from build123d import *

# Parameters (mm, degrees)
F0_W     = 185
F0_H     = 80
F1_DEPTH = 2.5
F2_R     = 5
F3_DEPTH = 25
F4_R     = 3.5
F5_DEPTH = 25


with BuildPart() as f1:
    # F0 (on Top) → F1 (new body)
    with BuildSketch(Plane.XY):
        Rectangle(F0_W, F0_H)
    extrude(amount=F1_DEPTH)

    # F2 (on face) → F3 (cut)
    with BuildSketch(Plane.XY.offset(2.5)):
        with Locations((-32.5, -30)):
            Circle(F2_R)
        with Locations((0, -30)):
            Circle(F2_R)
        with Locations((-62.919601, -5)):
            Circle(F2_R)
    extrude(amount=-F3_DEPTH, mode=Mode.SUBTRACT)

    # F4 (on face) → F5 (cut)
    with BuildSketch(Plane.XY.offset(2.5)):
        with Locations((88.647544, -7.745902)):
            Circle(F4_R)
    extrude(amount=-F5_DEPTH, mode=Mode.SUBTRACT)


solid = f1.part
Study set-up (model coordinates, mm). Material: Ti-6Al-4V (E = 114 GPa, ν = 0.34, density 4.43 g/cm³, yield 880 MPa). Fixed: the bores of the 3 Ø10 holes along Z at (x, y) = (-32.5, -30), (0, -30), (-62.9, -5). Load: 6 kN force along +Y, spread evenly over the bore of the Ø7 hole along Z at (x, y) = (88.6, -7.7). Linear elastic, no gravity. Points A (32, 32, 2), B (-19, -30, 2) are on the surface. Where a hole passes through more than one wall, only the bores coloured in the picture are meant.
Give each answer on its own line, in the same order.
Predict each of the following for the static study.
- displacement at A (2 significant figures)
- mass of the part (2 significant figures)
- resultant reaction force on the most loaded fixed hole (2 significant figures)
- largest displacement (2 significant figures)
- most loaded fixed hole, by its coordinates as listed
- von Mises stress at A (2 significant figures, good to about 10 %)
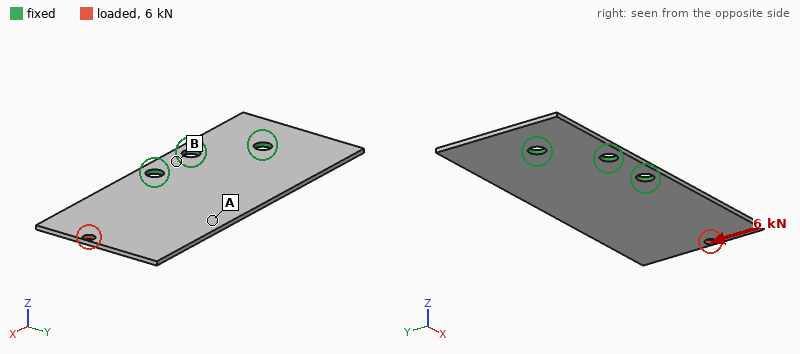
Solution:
0.16 mm
160 g
13 kN
0.36 mm
(0, -30)
100 MPa
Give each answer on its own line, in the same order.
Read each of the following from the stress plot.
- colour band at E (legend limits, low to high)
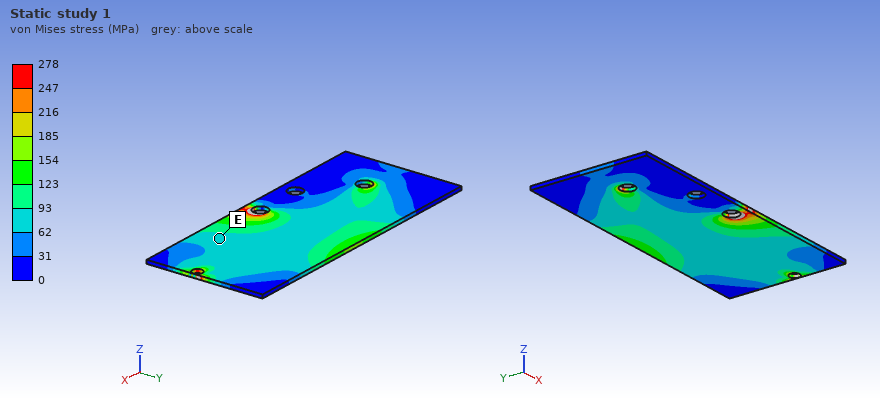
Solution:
62 to 93 MPa
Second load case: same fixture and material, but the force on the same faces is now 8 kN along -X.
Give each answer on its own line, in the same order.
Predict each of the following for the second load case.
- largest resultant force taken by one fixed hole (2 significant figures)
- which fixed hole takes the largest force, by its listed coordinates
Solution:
4.7 kN
(0, -30)
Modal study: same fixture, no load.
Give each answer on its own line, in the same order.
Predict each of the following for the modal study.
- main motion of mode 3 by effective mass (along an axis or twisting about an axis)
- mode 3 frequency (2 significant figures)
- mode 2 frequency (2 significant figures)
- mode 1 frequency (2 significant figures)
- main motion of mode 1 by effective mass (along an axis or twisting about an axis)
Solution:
along Z
880 Hz
460 Hz
200 Hz
along Z
